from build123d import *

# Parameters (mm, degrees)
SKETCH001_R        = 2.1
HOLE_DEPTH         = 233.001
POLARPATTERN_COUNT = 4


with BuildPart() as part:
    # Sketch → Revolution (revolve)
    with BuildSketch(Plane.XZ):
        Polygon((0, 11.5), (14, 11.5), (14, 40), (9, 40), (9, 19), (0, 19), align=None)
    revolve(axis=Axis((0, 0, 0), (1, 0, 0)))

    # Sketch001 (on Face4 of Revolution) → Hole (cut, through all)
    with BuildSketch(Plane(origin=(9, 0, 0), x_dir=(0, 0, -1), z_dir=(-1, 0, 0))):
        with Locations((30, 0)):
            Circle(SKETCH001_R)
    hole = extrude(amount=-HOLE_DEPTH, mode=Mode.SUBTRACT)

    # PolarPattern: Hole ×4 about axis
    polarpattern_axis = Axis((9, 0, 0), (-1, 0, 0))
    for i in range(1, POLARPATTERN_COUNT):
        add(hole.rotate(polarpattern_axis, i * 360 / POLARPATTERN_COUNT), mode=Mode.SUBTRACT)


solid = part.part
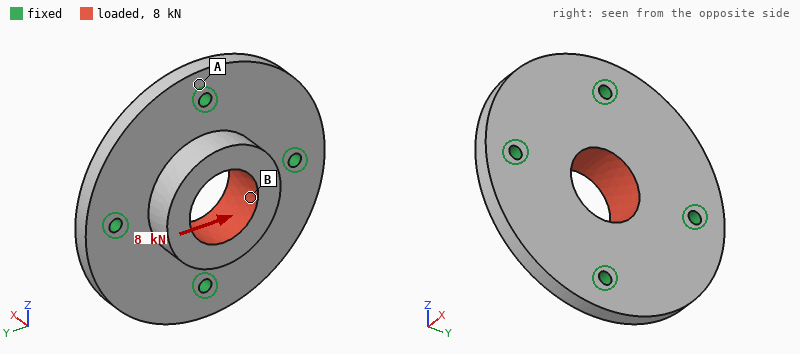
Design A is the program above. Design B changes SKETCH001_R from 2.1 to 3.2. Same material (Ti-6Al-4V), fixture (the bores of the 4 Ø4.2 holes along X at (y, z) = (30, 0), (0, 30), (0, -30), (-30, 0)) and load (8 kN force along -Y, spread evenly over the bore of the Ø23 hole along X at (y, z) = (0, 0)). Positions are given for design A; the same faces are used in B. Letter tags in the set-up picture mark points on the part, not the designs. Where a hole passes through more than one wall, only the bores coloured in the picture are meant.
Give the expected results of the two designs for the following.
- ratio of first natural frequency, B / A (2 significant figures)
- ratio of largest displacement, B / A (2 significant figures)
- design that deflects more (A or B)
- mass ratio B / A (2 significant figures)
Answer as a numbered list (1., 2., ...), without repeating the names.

1. 1.1
2. 0.85
3. A
4. 0.99
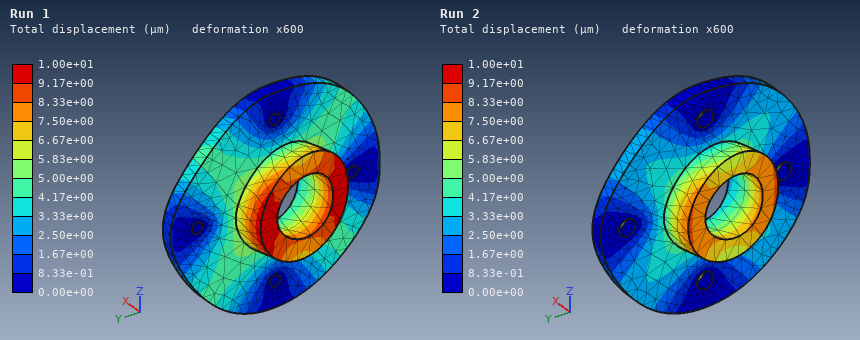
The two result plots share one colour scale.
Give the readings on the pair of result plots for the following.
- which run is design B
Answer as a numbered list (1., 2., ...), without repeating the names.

1. Run 2
